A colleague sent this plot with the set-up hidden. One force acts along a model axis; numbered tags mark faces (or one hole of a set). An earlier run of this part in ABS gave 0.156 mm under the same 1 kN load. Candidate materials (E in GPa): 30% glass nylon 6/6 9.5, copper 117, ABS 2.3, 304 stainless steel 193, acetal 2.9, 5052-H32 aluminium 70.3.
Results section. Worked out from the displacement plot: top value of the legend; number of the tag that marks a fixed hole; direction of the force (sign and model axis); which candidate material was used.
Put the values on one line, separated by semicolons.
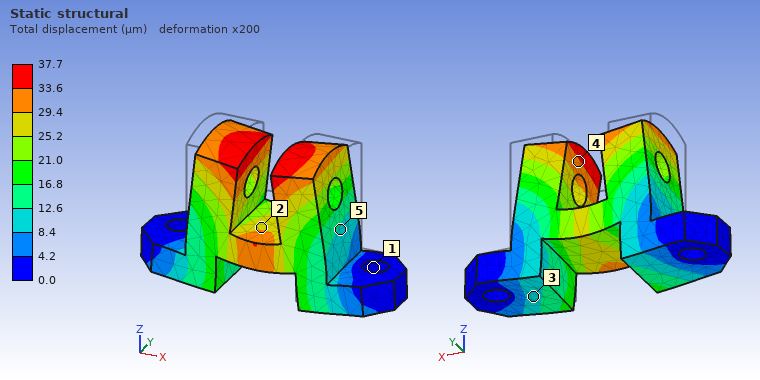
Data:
37.7 µm; 1; -Z; 30% glass nylon 6/6
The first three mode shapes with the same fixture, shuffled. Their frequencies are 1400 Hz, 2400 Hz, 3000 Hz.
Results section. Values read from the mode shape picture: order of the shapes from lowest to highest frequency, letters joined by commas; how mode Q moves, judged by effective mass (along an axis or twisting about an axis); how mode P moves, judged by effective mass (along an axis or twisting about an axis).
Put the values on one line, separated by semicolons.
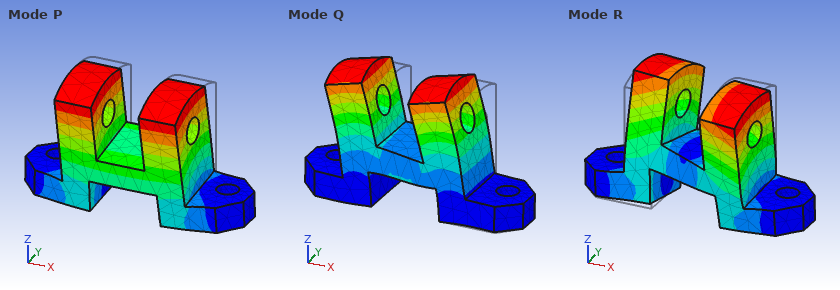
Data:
P, R, Q; along X; along Y
